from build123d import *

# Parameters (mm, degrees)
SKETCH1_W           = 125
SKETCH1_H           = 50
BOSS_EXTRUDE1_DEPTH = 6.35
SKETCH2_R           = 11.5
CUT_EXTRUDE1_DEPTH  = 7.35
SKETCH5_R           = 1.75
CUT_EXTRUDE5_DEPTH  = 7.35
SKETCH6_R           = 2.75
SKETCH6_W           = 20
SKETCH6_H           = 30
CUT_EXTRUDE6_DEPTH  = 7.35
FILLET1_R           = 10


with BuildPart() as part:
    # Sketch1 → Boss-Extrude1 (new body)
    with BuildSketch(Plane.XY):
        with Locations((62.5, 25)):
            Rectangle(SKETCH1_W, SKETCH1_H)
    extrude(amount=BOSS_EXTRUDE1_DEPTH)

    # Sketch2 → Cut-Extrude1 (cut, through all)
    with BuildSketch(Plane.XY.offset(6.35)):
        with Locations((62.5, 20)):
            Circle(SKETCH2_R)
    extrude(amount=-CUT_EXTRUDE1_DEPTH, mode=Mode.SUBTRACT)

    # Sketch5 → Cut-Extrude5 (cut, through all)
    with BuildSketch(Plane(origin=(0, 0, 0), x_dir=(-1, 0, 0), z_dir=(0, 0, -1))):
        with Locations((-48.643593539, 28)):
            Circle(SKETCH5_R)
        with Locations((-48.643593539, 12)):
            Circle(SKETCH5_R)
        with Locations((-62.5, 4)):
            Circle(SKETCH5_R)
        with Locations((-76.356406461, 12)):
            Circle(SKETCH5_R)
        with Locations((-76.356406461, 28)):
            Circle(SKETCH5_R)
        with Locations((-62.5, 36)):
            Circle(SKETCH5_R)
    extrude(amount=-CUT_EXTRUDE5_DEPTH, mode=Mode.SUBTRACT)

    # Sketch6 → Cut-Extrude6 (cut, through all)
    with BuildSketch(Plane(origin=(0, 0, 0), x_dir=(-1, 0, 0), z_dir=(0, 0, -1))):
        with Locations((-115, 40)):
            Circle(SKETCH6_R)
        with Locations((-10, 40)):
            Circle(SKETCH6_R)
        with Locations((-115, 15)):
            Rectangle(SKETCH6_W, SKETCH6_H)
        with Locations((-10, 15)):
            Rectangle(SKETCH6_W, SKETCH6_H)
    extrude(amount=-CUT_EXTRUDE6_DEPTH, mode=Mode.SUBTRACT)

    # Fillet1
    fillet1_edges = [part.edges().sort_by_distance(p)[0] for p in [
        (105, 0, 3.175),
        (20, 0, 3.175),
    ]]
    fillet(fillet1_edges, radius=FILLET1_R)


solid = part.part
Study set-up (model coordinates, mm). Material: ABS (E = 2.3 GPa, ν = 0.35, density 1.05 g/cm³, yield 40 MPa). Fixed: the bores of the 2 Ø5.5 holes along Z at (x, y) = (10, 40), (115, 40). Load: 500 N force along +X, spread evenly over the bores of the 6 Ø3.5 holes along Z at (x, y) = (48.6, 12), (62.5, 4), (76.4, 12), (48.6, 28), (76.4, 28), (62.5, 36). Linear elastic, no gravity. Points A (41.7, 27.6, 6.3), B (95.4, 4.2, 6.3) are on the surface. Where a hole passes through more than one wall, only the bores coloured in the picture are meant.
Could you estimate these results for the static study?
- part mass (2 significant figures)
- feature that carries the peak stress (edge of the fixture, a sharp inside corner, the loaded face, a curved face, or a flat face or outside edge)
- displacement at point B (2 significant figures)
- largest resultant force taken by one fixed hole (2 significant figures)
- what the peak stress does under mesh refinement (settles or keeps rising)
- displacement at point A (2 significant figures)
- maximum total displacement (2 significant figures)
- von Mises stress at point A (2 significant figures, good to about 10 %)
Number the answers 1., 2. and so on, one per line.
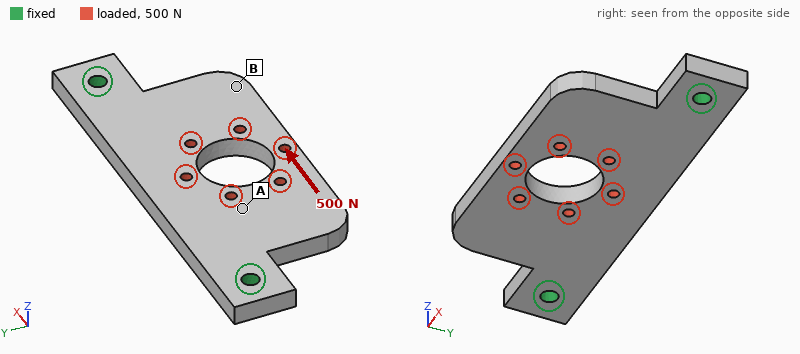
1. 30 g
2. edge of the fixture
3. 65 µm
4. 270 N
5. keeps rising
6. 33 µm
7. 72 µm
8. 1.5 MPa
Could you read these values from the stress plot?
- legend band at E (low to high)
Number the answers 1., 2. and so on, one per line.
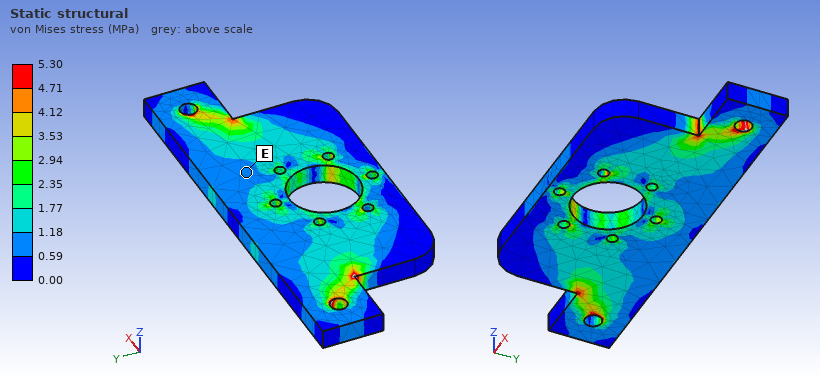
1. 0.59 to 1.18 MPa
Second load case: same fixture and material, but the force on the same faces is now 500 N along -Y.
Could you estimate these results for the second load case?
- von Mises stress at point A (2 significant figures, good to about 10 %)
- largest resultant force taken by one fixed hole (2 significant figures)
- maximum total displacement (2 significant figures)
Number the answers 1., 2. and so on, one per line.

1. 1.7 MPa
2. 290 N
3. 0.16 mm
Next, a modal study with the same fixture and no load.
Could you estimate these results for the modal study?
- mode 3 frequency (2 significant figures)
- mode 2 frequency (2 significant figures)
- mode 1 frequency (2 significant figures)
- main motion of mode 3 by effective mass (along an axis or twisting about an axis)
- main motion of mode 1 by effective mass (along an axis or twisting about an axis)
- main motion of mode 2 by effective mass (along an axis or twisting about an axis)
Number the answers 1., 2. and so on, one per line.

1. 1100 Hz
2. 970 Hz
3. 460 Hz
4. twisting about Y
5. along Z
6. along Z
